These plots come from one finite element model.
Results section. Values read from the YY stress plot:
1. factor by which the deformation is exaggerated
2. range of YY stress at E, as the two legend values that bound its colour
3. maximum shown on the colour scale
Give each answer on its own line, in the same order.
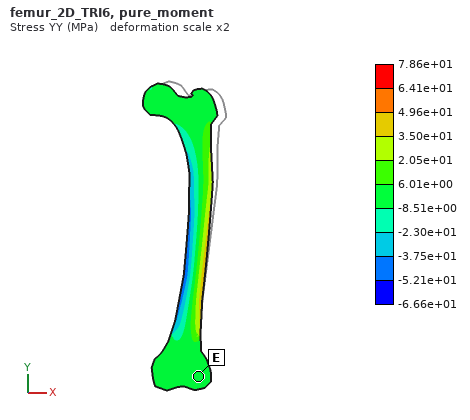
2
-8.51e+00 to 6.01e+00 MPa
7.86e+01 MPa
